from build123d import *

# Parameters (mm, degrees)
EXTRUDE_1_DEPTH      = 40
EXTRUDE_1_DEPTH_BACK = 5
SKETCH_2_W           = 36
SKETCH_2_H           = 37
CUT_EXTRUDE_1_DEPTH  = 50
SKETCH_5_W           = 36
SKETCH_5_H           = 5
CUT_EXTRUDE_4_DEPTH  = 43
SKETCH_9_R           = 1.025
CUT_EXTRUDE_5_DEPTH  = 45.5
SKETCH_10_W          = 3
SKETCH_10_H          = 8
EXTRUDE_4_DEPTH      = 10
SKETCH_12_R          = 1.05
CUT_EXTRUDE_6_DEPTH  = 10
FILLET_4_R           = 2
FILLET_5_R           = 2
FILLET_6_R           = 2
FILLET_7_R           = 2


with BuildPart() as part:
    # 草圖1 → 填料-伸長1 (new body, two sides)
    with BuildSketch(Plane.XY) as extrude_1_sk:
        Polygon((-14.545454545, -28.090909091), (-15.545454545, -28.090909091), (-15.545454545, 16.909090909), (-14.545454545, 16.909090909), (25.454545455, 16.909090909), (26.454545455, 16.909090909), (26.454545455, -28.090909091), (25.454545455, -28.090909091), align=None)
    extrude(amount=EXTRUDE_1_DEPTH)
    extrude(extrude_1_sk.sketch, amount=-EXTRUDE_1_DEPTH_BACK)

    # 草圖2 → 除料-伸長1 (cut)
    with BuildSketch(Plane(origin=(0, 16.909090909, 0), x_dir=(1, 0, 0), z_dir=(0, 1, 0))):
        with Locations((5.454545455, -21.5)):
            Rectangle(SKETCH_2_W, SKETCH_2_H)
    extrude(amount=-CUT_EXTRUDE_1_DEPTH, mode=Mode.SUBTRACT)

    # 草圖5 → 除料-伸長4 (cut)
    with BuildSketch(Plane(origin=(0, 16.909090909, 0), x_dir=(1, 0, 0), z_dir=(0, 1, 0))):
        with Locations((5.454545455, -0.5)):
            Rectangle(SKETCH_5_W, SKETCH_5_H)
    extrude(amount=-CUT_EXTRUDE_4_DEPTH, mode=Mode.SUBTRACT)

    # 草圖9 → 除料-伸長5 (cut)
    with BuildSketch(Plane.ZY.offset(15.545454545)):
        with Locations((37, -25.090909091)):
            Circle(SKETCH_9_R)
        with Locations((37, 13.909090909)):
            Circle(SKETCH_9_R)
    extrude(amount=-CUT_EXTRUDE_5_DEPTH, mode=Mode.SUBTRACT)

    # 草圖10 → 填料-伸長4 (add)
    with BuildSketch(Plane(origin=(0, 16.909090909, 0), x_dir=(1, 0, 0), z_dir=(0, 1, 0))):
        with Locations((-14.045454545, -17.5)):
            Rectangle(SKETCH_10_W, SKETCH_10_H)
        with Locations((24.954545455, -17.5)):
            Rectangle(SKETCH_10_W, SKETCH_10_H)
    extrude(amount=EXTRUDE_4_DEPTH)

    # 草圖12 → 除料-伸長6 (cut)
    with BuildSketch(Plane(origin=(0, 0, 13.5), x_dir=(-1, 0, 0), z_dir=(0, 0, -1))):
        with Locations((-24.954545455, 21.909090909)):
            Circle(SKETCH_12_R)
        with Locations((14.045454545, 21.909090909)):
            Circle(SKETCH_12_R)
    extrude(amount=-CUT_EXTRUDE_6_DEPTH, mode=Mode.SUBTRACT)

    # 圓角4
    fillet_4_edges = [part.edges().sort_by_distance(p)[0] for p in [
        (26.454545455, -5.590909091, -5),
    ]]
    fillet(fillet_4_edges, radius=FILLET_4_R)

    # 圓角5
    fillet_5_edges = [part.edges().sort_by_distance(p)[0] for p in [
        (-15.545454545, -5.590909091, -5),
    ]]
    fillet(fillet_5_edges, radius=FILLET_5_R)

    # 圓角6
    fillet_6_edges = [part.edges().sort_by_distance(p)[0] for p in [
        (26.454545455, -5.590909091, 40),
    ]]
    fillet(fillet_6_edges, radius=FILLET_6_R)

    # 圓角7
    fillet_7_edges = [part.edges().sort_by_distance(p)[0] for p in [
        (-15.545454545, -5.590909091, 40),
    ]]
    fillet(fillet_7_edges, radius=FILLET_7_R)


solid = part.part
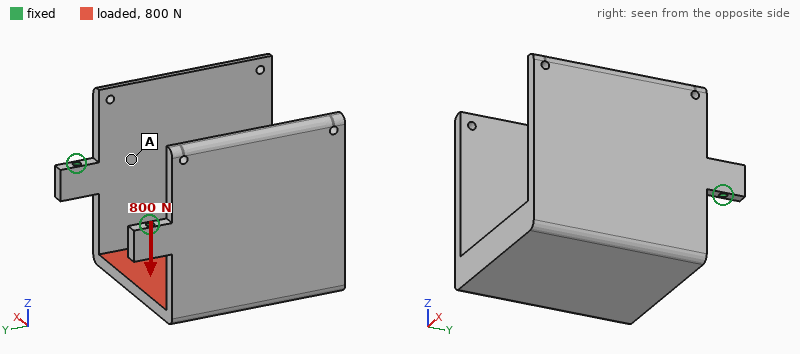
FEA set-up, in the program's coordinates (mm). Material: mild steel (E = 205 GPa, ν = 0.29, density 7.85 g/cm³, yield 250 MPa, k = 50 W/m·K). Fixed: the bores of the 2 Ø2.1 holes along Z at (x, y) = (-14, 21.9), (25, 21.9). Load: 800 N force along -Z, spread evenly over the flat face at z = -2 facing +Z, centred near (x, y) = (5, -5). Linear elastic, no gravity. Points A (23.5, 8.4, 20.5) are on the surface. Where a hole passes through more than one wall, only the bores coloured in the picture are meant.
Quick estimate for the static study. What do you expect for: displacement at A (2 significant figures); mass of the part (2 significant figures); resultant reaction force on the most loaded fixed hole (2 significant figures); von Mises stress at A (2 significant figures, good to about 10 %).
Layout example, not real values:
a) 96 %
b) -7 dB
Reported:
a) 0.027 mm
b) 140 g
c) 400 N
d) 33 MPa
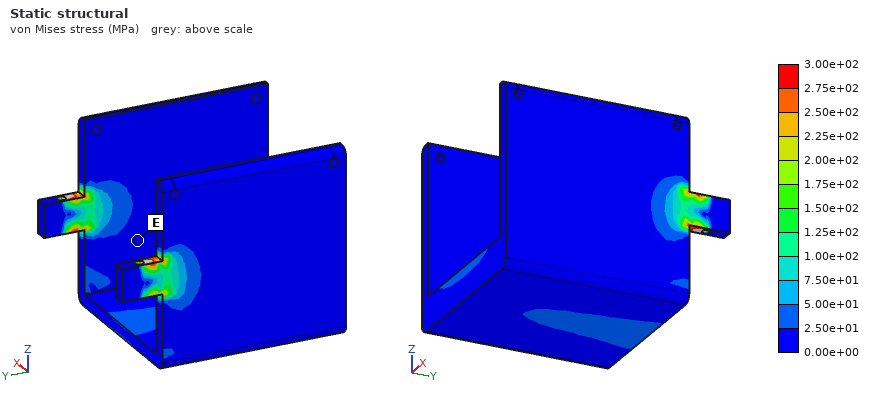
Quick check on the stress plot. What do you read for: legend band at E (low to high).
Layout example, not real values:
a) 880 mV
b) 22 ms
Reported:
a) 0.00e+00 to 2.50e+01 MPa
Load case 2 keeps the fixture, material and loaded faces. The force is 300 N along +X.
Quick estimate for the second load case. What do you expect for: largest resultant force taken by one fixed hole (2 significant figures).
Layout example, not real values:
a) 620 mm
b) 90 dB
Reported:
a) 230 N
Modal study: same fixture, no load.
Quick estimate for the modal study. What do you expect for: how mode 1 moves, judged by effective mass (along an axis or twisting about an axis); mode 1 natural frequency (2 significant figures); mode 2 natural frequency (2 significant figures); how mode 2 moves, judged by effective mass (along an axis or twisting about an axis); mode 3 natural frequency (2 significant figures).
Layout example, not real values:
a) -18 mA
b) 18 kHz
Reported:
a) along X
b) 1000 Hz
c) 1200 Hz
d) along Z
e) 1700 Hz
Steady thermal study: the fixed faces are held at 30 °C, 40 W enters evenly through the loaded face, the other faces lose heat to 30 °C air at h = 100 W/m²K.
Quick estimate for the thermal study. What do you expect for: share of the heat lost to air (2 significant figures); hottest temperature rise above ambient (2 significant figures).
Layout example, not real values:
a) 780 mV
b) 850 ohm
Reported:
a) 86 %
b) 69 K
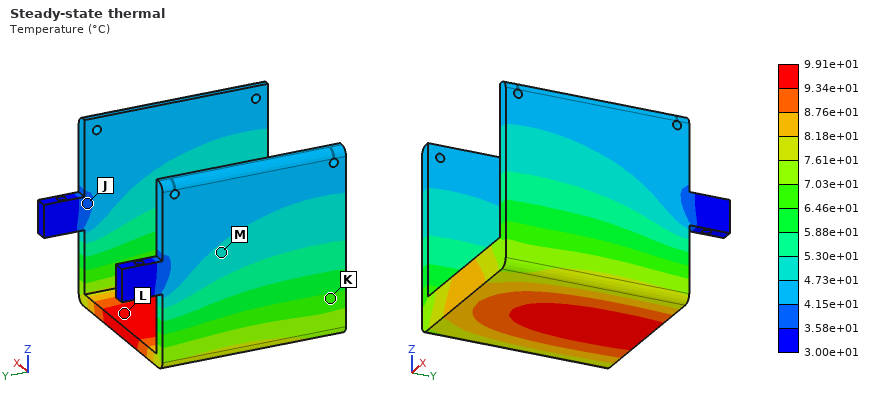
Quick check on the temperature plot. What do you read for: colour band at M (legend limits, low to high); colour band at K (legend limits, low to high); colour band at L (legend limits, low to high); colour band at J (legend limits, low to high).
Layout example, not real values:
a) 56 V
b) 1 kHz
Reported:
a) 4.73e+01 to 5.30e+01 °C
b) 6.46e+01 to 7.03e+01 °C
c) 9.34e+01 to 9.91e+01 °C
d) 3.58e+01 to 4.15e+01 °C
